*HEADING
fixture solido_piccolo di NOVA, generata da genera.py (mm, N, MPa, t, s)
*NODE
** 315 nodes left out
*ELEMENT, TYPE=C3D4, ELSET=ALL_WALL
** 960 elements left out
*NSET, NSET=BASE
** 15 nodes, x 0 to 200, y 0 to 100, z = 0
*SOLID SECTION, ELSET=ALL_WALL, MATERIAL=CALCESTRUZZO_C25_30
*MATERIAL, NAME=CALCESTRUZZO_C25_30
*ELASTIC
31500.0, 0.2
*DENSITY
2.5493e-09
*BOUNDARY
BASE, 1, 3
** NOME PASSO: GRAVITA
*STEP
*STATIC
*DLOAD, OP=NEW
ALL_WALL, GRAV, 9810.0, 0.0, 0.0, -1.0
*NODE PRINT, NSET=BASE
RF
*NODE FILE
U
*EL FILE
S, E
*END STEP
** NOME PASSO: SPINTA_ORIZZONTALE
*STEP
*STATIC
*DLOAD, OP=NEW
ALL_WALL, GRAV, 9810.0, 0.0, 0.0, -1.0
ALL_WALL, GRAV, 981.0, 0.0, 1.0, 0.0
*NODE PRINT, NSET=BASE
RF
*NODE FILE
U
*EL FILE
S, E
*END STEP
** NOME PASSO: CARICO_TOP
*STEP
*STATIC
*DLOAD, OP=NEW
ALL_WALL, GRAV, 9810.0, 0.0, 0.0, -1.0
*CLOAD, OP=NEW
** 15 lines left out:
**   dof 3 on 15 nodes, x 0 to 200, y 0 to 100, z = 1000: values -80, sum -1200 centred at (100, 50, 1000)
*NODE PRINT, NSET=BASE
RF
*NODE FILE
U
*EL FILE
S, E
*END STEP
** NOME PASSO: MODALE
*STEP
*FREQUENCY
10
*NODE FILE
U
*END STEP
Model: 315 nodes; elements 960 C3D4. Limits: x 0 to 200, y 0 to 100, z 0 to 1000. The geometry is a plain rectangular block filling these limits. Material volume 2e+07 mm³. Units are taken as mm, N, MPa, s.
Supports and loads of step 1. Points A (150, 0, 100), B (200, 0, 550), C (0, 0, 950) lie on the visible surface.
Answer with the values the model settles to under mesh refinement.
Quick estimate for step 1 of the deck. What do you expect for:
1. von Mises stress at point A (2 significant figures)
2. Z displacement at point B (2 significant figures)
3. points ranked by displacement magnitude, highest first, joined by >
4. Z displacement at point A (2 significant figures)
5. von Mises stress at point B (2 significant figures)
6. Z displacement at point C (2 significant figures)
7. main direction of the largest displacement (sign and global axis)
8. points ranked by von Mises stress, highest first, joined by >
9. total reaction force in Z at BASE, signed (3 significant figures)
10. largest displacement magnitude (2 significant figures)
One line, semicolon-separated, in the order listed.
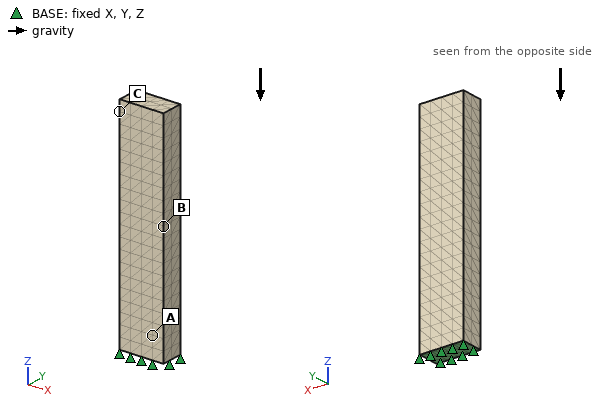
0.023 MPa; -3.1e-04 mm; C > B > A; -7.4e-05 mm; 0.011 MPa; -3.9e-04 mm; -Z; A > B > C; 500 N; 4.0e-04 mm
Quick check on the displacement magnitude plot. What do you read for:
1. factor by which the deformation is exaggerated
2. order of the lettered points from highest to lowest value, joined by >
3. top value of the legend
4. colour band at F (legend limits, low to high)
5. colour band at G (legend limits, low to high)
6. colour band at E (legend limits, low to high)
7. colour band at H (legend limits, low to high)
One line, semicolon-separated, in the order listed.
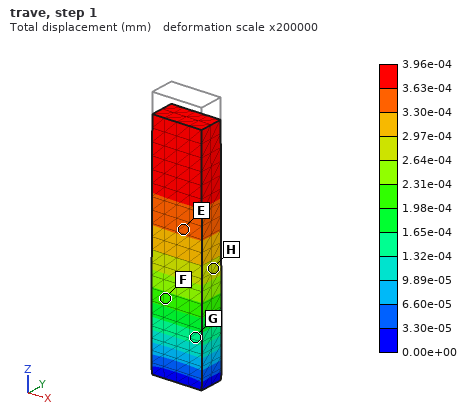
200000; E > H > F > G; 3.96e-04 mm; 1.98e-04 to 2.31e-04 mm; 1.32e-04 to 1.65e-04 mm; 3.30e-04 to 3.63e-04 mm; 2.64e-04 to 2.97e-04 mm
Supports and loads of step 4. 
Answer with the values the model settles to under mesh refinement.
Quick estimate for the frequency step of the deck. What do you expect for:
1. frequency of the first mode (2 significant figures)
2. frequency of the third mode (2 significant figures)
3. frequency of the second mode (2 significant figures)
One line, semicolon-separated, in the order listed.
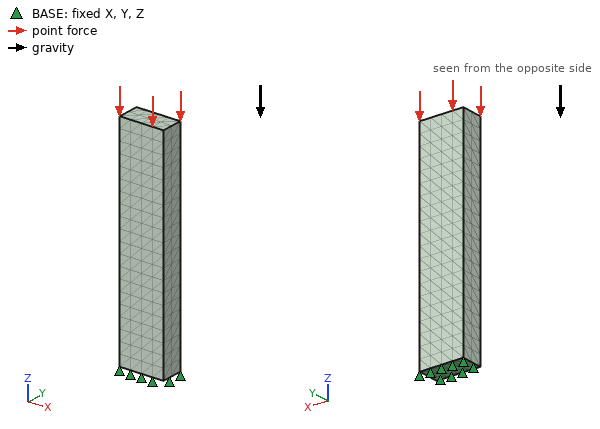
57 Hz; 340 Hz; 110 Hz
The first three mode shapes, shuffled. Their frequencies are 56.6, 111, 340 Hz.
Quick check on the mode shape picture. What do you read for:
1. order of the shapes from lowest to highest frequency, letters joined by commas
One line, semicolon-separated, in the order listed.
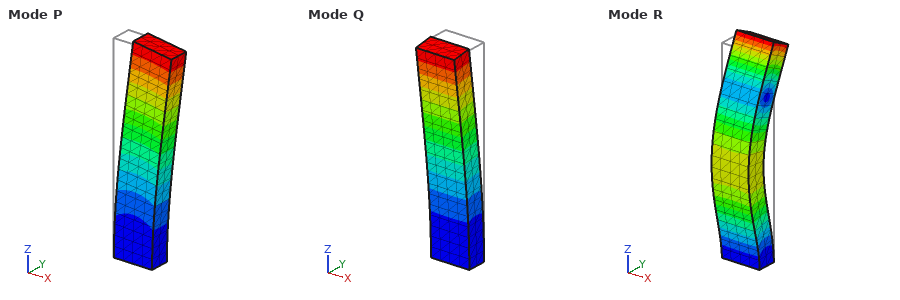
Q, P, R
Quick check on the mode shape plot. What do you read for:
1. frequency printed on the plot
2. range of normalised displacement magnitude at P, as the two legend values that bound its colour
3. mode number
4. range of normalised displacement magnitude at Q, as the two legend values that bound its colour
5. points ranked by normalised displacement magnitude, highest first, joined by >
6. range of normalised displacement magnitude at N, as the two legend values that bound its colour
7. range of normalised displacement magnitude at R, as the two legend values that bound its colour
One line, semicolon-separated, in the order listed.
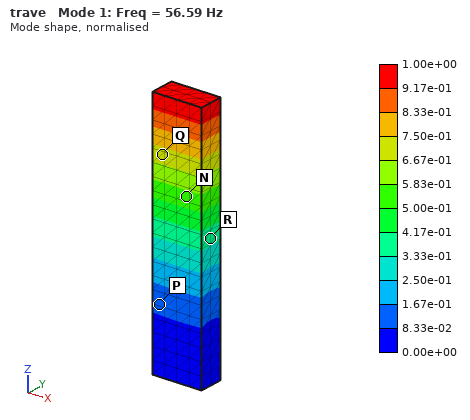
56.59 Hz; 8.33e-02 to 1.67e-01; 1; 6.67e-01 to 7.50e-01; Q > N > R > P; 5.00e-01 to 5.83e-01; 3.33e-01 to 4.17e-01
